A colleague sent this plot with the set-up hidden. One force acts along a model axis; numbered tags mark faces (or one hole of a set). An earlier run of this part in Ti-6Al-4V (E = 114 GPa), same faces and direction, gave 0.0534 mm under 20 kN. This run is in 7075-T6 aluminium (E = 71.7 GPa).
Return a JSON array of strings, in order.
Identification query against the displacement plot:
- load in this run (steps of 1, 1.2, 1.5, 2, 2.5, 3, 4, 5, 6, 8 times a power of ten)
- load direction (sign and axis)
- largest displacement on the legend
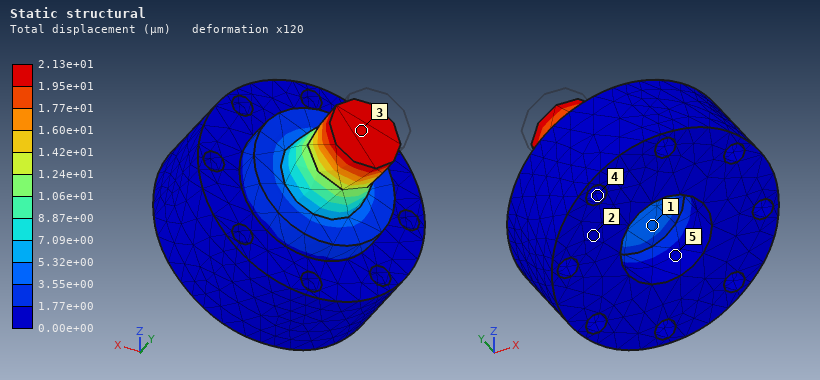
["5 kN", "-Y", "2.13e+01 µm"]
